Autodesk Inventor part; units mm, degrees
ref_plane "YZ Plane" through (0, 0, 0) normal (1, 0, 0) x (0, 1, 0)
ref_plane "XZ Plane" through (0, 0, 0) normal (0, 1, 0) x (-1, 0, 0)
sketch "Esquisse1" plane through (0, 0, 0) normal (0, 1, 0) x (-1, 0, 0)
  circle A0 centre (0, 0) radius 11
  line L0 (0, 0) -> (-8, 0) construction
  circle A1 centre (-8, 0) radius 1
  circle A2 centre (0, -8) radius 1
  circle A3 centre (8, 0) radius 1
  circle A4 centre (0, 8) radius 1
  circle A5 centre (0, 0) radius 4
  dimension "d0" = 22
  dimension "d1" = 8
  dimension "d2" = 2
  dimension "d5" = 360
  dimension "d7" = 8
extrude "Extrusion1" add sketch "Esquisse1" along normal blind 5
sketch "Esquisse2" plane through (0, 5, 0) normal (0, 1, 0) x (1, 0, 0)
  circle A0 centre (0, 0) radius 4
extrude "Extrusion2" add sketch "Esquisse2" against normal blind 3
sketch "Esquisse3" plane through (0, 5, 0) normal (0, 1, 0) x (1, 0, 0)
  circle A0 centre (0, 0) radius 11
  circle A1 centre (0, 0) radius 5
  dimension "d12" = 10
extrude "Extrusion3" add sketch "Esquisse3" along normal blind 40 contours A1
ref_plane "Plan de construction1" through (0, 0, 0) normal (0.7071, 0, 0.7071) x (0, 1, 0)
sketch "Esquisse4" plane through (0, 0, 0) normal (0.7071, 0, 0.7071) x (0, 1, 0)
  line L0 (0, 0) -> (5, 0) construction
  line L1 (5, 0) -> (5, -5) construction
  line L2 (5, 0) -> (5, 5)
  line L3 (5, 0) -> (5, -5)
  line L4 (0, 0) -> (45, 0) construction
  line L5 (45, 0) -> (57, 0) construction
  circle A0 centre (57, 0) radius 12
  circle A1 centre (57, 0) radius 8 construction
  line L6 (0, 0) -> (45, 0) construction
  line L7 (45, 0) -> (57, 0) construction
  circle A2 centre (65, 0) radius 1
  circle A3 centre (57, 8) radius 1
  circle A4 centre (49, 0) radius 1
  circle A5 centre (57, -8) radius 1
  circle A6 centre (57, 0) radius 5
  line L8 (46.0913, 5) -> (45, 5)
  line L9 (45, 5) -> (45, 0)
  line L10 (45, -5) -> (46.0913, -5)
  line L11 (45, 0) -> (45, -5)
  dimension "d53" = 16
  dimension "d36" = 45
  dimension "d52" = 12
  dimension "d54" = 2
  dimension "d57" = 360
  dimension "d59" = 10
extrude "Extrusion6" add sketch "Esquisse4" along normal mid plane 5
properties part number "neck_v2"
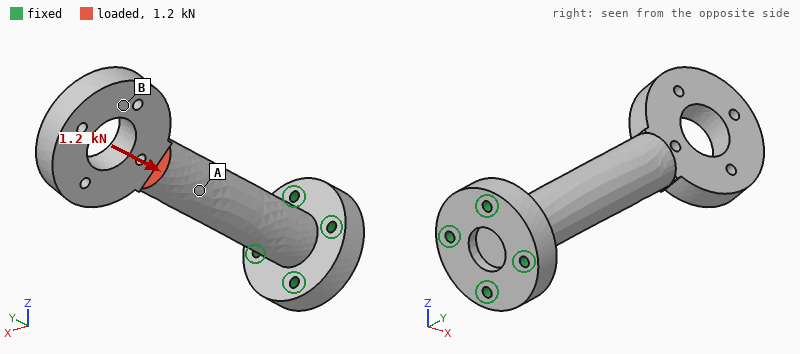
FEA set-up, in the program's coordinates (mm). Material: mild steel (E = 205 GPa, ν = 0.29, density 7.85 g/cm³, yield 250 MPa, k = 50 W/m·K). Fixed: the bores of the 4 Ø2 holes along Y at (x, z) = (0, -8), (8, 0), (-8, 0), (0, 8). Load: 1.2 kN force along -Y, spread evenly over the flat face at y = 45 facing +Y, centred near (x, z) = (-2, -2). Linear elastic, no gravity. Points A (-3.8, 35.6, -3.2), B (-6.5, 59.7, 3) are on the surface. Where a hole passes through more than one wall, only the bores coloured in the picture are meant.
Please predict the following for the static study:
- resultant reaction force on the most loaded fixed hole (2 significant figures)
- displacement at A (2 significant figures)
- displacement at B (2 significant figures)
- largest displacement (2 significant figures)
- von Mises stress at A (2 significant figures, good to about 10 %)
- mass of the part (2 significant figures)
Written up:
520 N
26 µm
66 µm
83 µm
59 MPa
53 g
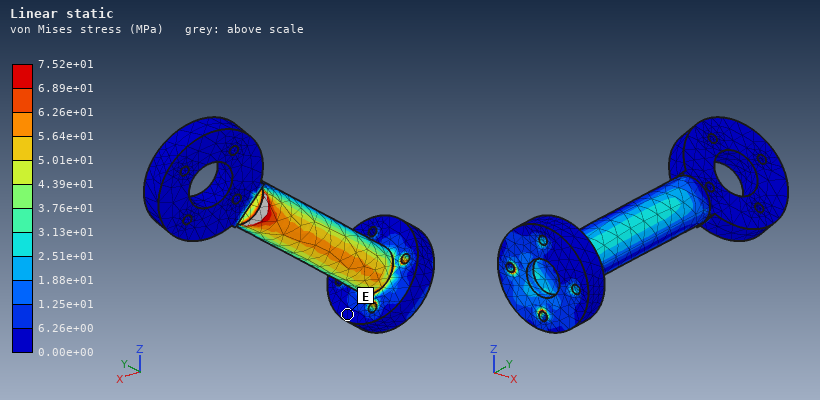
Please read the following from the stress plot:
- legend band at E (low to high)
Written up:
0.00e+00 to 6.26e+00 MPa
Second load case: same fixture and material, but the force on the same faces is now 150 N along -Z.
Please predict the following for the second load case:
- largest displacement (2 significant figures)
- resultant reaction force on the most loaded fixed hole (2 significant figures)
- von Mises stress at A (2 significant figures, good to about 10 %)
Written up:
75 µm
430 N
11 MPa
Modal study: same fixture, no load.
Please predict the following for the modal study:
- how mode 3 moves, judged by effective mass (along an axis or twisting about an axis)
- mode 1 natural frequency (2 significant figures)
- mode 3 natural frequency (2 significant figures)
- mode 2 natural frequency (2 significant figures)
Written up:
twisting about Y
1600 Hz
6700 Hz
1600 Hz
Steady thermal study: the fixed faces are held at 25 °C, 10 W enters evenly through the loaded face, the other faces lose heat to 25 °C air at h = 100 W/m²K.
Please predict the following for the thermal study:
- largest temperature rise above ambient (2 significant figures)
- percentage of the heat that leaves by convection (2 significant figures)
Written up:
70 K
68 %
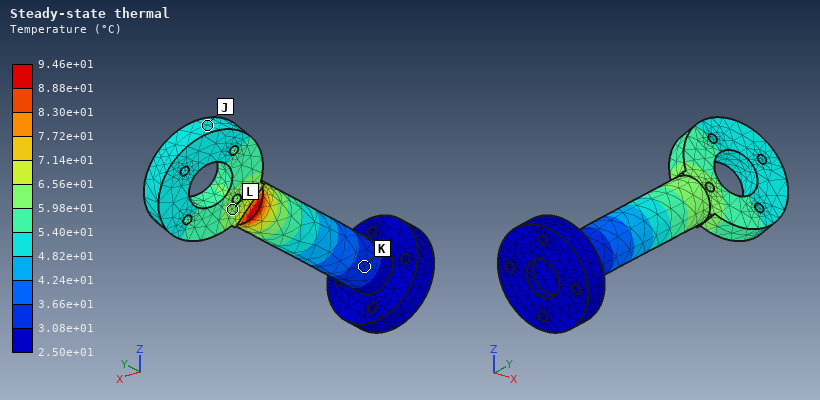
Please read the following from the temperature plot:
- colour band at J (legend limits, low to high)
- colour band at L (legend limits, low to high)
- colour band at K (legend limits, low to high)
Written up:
4.82e+01 to 5.40e+01 °C
5.98e+01 to 6.56e+01 °C
3.08e+01 to 3.66e+01 °C
